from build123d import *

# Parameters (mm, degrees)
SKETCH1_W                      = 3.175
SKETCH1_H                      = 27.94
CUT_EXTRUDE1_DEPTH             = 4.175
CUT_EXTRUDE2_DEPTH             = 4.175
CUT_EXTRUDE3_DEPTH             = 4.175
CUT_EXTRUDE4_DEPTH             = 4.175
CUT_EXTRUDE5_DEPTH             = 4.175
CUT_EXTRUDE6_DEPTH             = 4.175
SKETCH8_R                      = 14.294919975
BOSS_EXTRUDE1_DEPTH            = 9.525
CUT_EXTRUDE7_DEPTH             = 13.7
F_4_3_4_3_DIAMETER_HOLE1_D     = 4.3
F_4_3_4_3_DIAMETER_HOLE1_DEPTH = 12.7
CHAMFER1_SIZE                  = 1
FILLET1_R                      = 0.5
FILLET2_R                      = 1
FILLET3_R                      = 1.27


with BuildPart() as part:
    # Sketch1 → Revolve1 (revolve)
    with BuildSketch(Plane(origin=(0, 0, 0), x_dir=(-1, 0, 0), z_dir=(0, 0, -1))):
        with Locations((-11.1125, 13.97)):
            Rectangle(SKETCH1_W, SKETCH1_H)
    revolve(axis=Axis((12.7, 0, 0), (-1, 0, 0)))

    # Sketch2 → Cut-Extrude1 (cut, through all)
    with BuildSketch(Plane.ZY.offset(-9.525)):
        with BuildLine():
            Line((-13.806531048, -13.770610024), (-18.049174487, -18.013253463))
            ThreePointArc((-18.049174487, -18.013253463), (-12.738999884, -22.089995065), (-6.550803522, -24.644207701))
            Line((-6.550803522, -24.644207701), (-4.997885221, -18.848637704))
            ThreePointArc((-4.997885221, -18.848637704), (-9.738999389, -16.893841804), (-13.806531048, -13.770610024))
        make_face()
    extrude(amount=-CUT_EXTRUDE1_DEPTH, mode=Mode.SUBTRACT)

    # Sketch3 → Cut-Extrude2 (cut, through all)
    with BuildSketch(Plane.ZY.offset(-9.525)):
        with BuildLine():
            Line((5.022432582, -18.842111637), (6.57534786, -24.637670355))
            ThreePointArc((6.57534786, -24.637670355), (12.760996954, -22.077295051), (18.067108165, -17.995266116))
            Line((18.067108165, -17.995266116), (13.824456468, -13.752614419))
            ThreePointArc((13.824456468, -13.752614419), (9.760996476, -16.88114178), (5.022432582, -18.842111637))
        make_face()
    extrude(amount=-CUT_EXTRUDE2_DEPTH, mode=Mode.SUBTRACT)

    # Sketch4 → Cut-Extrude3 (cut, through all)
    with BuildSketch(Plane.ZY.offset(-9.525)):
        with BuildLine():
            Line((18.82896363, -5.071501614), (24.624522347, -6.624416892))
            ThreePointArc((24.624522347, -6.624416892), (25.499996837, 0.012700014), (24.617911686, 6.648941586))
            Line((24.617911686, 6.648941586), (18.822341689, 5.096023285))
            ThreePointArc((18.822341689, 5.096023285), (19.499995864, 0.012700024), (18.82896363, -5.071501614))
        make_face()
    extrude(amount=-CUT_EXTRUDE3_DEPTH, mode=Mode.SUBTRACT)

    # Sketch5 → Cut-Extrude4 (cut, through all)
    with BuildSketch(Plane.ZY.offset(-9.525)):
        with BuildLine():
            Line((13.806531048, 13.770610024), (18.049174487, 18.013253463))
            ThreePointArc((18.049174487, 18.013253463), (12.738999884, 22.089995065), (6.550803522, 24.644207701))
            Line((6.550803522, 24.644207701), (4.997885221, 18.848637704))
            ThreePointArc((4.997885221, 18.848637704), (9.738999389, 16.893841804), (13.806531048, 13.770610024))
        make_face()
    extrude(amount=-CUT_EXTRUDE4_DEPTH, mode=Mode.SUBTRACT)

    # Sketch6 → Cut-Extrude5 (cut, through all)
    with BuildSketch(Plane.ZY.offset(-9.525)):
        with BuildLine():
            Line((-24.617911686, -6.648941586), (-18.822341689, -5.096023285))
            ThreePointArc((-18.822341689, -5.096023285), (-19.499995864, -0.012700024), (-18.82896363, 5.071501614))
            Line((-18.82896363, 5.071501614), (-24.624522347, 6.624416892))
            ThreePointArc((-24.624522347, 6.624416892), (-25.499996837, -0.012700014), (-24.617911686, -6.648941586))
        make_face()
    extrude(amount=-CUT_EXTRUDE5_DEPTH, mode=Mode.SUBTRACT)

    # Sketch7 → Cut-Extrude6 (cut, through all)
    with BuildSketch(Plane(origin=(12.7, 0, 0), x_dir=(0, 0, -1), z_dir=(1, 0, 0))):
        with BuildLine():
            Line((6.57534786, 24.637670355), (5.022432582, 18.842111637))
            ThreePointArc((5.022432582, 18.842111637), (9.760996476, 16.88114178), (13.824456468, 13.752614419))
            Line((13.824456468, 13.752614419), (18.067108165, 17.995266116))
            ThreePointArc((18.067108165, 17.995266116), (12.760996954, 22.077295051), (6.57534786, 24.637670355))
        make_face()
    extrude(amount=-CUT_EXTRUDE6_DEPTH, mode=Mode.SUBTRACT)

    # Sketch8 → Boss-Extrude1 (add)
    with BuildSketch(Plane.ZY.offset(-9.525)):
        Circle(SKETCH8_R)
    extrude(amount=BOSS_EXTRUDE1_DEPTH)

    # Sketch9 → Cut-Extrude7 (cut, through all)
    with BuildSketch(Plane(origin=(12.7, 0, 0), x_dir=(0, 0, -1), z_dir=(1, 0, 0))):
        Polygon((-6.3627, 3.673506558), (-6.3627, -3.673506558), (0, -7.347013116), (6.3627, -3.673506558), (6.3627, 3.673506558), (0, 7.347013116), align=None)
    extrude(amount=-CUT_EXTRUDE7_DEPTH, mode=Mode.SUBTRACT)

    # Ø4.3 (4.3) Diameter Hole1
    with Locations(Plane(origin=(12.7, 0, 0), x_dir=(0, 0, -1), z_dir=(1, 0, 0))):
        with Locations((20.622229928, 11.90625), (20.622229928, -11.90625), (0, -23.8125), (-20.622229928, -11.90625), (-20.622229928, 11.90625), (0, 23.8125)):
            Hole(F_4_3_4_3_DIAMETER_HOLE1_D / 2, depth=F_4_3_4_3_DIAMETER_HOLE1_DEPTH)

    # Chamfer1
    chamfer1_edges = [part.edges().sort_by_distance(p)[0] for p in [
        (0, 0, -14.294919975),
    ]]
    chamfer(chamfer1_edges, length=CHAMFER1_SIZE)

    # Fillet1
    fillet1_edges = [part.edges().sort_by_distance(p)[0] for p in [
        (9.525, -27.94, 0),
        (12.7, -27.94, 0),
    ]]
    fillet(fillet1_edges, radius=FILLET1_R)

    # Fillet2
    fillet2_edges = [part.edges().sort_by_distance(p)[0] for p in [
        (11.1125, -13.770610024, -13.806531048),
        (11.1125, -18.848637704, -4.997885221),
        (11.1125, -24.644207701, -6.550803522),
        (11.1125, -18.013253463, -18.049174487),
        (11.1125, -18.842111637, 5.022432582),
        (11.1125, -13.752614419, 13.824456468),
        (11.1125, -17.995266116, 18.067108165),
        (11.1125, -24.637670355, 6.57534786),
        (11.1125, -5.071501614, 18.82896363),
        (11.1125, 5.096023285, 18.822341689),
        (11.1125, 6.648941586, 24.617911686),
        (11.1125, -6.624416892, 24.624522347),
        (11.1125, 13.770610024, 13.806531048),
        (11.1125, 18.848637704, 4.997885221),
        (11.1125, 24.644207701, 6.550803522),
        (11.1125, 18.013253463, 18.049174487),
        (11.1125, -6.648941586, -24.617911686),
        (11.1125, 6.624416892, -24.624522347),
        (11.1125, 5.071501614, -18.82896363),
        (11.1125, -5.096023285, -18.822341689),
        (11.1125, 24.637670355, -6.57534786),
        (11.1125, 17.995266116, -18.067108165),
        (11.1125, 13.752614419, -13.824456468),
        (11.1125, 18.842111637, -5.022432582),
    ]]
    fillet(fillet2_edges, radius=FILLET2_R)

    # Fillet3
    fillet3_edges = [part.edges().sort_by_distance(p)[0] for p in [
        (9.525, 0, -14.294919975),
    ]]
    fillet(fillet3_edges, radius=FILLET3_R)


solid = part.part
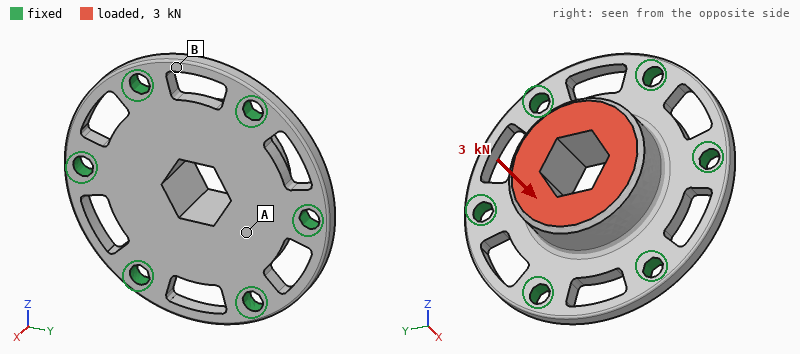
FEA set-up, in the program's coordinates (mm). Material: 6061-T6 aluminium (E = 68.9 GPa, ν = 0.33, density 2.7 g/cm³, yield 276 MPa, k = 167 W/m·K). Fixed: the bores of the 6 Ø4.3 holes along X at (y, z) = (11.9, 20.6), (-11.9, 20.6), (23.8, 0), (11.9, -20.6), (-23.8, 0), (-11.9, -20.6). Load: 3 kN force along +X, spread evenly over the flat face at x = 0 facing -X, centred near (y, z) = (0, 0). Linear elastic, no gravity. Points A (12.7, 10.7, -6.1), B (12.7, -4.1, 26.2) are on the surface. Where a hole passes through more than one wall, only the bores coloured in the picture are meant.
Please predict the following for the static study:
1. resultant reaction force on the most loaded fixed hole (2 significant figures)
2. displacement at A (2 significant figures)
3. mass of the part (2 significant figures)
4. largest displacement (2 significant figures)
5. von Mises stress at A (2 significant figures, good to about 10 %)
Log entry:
580 N
22 µm
28 g
24 µm
25 MPa
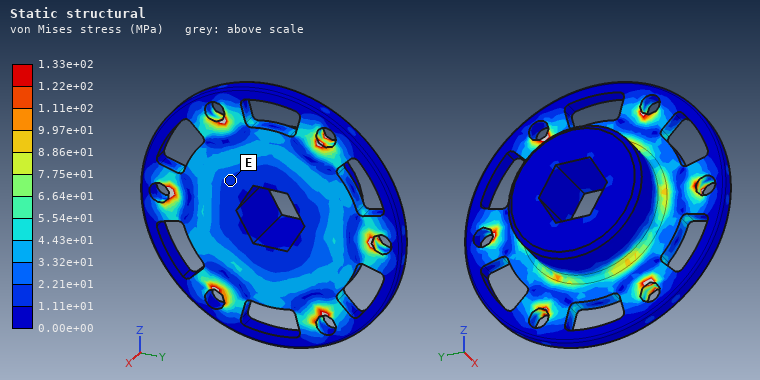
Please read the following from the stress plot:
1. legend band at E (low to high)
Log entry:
1.11e+01 to 2.21e+01 MPa
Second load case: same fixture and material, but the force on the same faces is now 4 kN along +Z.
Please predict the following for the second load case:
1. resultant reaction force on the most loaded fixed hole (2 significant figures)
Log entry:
1.1 kN
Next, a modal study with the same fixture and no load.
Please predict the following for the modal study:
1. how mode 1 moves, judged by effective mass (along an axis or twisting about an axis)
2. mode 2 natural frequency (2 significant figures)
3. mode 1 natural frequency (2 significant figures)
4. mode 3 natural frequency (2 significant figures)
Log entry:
along X
18 kHz
13 kHz
18 kHz
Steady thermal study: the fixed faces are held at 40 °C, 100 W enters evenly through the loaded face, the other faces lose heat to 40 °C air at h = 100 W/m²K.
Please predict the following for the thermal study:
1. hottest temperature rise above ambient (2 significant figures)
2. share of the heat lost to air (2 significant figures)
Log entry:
37 K
8.2 %
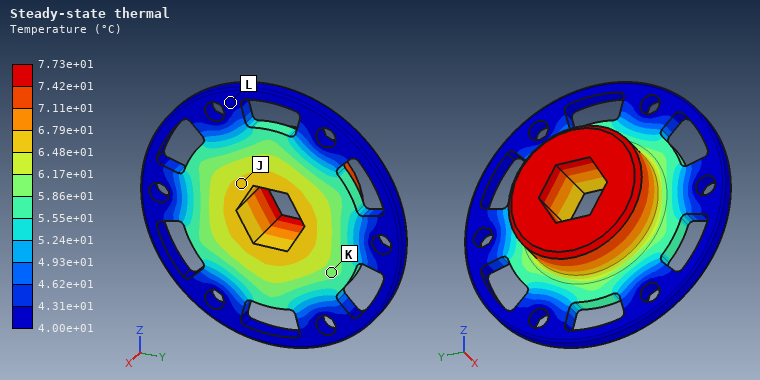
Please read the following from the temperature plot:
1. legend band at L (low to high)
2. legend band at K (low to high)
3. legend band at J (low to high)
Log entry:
4.00e+01 to 4.31e+01 °C
5.86e+01 to 6.17e+01 °C
6.48e+01 to 6.79e+01 °C
